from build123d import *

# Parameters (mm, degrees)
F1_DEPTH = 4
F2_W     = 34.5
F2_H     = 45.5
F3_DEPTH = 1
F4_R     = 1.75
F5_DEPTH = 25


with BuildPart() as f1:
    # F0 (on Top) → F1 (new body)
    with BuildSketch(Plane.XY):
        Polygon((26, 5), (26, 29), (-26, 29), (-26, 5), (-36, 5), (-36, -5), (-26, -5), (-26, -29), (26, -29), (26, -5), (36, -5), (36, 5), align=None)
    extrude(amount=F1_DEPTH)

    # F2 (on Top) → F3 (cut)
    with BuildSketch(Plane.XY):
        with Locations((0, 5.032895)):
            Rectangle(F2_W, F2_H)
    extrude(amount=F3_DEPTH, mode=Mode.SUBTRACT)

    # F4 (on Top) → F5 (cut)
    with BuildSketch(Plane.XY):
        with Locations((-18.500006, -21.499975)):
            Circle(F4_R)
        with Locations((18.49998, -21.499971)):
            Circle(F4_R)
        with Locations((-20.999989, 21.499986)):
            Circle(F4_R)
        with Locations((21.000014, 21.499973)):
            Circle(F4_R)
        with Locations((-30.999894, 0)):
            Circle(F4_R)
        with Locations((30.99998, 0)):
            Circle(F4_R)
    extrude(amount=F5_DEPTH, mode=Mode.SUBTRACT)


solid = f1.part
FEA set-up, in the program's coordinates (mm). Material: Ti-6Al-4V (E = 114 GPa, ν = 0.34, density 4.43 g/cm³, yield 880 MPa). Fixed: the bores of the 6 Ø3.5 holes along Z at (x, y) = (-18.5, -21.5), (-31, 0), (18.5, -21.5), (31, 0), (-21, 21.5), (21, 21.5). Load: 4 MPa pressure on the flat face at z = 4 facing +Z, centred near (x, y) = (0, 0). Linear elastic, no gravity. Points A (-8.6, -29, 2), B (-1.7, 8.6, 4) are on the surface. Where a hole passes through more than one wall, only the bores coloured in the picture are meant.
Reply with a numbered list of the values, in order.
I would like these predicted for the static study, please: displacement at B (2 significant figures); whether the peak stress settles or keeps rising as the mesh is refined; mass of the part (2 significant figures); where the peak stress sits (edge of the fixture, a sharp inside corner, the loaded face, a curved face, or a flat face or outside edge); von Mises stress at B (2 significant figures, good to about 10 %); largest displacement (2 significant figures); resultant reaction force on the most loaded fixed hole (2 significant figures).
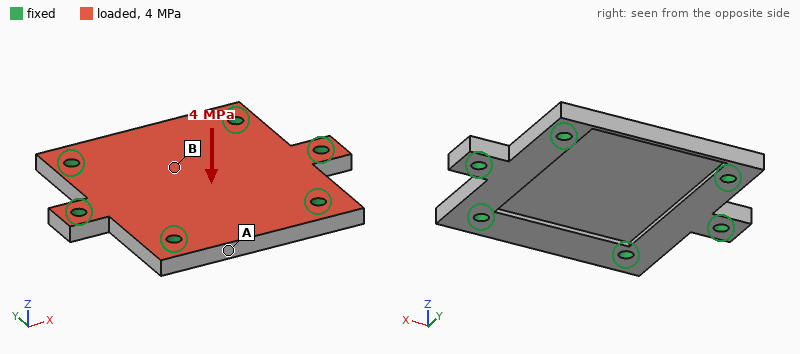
1. 0.16 mm
2. keeps rising
3. 49 g
4. edge of the fixture
5. 180 MPa
6. 0.17 mm
7. 2.6 kN
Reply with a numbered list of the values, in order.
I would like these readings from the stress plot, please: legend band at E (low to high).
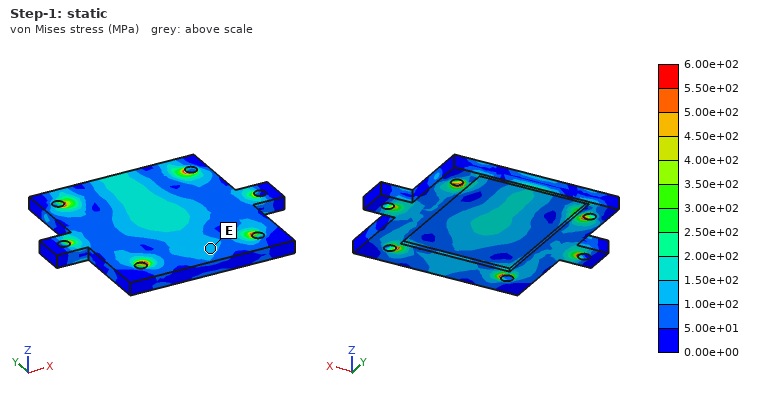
1. 1.00e+02 to 1.50e+02 MPa
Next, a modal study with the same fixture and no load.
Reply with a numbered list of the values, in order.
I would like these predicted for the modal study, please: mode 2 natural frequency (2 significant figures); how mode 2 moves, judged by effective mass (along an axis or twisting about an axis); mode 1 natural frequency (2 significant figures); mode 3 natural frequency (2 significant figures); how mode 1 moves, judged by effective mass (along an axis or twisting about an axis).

1. 12 kHz
2. twisting about X
3. 8300 Hz
4. 15 kHz
5. along Z
